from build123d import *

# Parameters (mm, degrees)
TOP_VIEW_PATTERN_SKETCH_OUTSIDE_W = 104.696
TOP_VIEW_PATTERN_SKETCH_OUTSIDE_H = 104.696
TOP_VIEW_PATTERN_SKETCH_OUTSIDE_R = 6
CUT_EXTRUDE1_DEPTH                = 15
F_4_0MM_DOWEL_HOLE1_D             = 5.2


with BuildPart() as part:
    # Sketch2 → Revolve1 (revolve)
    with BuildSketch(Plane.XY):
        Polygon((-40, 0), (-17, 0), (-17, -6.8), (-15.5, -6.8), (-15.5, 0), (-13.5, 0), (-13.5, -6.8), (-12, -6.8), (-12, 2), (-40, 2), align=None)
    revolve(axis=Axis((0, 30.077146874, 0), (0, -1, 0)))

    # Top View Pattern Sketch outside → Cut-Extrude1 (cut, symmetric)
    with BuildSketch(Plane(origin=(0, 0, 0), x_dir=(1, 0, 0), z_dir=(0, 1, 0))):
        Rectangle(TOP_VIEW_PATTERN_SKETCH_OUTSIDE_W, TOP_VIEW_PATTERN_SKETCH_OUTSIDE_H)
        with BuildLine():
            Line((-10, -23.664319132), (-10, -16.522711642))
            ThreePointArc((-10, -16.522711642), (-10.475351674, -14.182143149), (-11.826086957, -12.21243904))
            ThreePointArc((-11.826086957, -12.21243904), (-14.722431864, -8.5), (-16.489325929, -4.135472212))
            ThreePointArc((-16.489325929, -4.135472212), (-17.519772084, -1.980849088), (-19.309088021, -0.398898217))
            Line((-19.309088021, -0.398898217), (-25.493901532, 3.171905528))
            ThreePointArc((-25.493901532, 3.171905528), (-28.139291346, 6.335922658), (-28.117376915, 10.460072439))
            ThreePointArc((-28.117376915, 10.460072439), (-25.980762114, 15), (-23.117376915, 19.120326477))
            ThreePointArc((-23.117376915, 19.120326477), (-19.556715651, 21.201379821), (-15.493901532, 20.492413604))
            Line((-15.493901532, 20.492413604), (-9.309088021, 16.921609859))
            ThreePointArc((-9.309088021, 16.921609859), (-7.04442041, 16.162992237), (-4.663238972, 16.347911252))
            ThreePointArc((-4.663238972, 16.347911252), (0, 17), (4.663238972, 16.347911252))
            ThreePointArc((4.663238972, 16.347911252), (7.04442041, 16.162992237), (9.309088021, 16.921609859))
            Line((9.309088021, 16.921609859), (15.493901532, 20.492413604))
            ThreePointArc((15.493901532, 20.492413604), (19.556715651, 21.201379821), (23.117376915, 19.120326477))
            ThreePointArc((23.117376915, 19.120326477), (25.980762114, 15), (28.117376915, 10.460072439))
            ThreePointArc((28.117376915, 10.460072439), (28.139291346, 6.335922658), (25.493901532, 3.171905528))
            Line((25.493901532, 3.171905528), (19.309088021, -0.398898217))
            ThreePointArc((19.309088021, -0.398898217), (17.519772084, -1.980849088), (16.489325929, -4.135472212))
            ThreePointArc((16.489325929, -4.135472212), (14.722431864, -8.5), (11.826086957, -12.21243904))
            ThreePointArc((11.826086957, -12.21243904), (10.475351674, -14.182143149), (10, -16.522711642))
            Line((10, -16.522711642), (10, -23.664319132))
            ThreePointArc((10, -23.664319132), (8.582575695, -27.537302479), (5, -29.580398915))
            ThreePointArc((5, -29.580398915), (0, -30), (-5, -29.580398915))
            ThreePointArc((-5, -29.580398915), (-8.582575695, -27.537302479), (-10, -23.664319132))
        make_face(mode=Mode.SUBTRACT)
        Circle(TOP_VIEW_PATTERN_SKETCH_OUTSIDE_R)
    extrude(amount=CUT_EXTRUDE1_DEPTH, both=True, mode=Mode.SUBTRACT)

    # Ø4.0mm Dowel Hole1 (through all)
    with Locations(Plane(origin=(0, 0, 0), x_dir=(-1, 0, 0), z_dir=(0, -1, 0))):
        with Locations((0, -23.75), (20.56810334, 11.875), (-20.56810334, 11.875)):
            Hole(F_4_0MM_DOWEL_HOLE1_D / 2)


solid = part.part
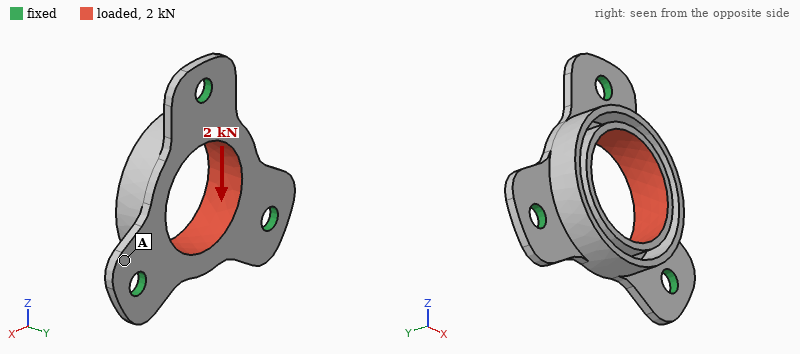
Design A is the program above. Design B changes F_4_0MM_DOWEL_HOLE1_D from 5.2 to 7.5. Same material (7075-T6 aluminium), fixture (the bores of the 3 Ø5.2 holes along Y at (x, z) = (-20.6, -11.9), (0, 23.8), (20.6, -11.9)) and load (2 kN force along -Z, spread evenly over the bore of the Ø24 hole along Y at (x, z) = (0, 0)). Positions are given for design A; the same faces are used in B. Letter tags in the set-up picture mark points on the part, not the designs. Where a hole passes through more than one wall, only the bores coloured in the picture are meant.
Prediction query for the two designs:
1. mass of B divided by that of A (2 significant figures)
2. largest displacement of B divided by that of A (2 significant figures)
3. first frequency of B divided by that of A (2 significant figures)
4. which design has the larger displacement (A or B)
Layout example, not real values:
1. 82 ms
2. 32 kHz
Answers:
1. 0.97
2. 0.76
3. 1.2
4. A
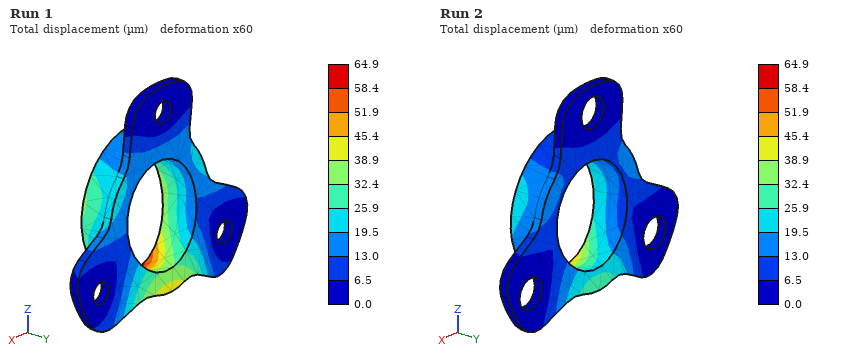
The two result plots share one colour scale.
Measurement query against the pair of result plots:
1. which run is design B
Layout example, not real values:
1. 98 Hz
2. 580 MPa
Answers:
1. Run 2
